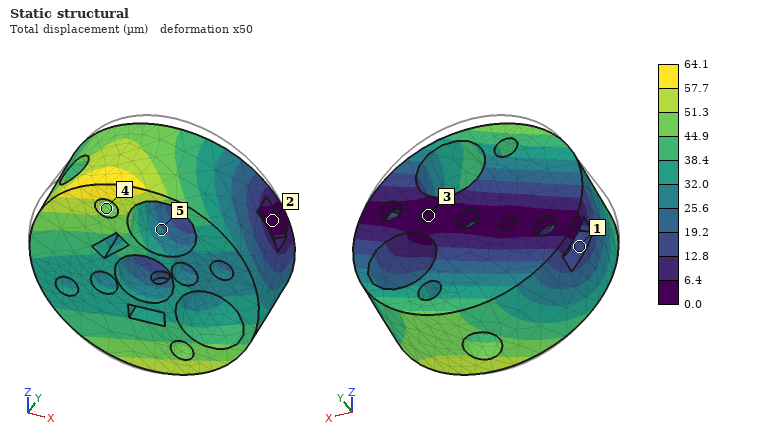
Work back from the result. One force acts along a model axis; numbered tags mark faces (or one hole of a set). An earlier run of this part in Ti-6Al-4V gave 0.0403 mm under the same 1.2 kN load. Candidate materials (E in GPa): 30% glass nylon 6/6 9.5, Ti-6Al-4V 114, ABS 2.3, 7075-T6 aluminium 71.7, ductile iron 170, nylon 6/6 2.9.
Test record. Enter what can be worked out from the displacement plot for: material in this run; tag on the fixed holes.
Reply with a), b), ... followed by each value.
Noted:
a) 7075-T6 aluminium
b) 3
